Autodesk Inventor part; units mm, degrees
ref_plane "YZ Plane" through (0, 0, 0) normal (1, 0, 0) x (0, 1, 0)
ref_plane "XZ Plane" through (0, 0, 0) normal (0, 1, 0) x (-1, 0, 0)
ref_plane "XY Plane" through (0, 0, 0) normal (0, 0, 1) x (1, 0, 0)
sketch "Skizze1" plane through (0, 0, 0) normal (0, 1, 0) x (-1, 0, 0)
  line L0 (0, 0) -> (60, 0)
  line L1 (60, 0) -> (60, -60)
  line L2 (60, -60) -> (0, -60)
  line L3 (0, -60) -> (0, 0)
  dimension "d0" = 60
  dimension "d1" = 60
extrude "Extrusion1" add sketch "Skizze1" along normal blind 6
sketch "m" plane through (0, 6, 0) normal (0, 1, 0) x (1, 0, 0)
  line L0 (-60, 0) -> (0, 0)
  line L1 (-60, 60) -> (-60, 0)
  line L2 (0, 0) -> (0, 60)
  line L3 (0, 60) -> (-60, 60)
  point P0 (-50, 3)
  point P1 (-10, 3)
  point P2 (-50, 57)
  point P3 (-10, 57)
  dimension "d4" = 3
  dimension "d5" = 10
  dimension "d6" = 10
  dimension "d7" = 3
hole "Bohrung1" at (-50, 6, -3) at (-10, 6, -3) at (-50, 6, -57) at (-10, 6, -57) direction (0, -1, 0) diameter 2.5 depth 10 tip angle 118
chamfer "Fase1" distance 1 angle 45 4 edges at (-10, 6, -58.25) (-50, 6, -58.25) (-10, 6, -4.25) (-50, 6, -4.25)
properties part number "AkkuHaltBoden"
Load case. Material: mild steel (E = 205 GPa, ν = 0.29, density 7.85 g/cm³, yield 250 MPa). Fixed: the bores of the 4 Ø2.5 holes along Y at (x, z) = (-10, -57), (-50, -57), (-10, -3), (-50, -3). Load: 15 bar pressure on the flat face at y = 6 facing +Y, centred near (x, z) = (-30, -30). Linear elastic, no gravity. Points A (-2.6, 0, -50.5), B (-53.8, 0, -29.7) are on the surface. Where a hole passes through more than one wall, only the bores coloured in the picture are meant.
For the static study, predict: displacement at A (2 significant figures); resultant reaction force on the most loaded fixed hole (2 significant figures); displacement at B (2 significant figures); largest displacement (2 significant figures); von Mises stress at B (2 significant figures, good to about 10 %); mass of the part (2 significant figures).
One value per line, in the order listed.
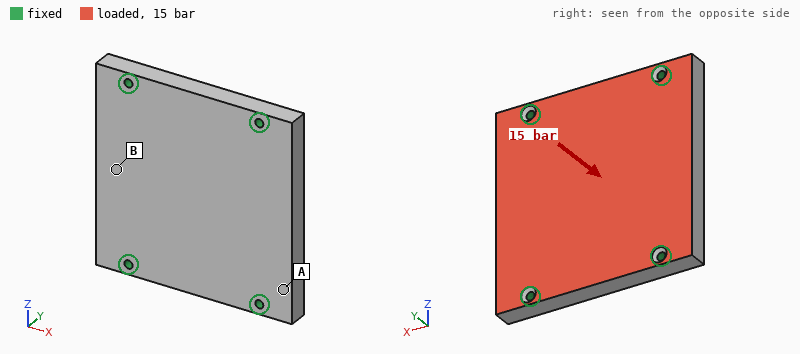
6.2 µm
1.3 kN
19 µm
22 µm
44 MPa
170 g
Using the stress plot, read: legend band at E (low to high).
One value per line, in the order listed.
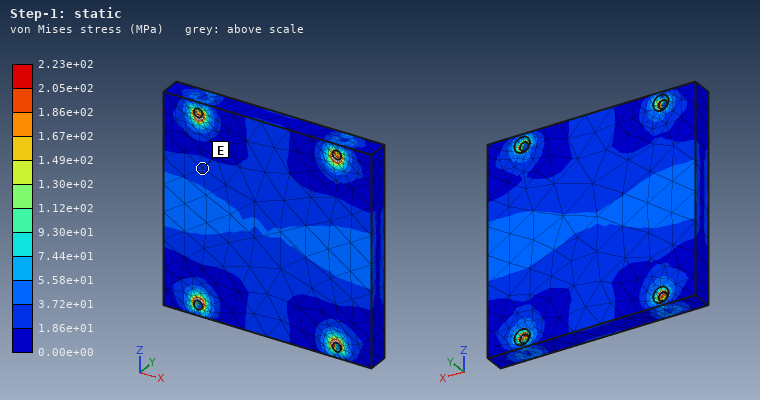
1.86e+01 to 3.72e+01 MPa
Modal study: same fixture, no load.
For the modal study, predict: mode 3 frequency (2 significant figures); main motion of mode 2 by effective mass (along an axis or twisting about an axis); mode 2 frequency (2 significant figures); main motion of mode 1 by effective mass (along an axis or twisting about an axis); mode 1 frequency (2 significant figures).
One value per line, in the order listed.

12 kHz
twisting about Z
9400 Hz
along Y
7000 Hz
